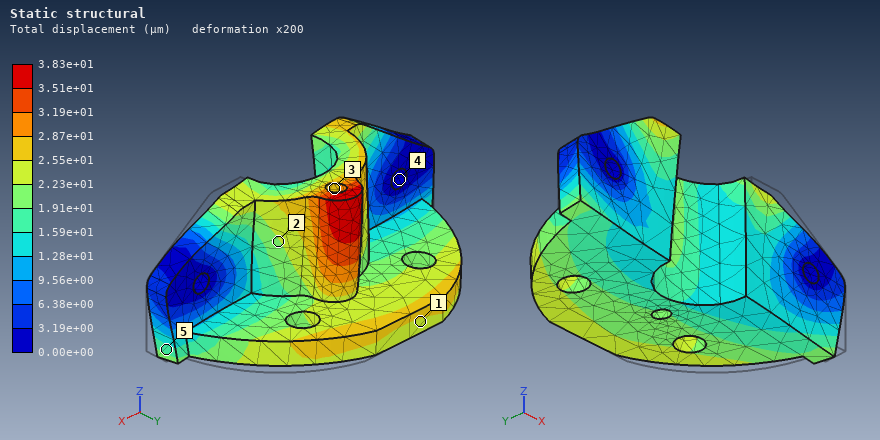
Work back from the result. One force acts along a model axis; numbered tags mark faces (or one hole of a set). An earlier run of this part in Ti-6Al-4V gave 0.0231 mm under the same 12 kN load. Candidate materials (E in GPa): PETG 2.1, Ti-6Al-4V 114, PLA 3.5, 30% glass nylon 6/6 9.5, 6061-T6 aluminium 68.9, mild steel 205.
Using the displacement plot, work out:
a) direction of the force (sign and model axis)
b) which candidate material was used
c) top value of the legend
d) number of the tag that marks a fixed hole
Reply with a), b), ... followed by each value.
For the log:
a) -X
b) 6061-T6 aluminium
c) 3.83e+01 µm
d) 4
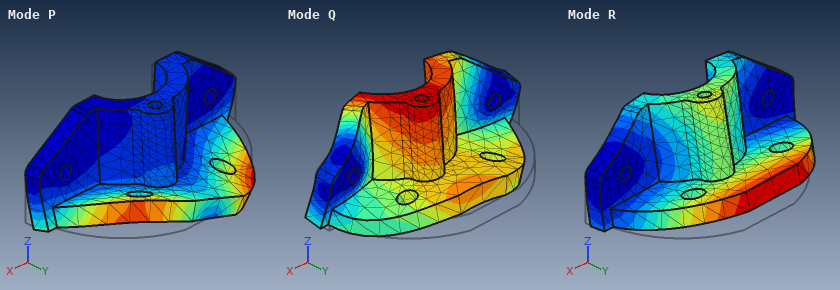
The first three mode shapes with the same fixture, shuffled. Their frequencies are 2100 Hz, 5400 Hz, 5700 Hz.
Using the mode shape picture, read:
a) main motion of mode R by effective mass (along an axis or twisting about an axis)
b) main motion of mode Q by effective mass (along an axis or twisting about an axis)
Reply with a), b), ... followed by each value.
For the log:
a) along Z
b) along Y
